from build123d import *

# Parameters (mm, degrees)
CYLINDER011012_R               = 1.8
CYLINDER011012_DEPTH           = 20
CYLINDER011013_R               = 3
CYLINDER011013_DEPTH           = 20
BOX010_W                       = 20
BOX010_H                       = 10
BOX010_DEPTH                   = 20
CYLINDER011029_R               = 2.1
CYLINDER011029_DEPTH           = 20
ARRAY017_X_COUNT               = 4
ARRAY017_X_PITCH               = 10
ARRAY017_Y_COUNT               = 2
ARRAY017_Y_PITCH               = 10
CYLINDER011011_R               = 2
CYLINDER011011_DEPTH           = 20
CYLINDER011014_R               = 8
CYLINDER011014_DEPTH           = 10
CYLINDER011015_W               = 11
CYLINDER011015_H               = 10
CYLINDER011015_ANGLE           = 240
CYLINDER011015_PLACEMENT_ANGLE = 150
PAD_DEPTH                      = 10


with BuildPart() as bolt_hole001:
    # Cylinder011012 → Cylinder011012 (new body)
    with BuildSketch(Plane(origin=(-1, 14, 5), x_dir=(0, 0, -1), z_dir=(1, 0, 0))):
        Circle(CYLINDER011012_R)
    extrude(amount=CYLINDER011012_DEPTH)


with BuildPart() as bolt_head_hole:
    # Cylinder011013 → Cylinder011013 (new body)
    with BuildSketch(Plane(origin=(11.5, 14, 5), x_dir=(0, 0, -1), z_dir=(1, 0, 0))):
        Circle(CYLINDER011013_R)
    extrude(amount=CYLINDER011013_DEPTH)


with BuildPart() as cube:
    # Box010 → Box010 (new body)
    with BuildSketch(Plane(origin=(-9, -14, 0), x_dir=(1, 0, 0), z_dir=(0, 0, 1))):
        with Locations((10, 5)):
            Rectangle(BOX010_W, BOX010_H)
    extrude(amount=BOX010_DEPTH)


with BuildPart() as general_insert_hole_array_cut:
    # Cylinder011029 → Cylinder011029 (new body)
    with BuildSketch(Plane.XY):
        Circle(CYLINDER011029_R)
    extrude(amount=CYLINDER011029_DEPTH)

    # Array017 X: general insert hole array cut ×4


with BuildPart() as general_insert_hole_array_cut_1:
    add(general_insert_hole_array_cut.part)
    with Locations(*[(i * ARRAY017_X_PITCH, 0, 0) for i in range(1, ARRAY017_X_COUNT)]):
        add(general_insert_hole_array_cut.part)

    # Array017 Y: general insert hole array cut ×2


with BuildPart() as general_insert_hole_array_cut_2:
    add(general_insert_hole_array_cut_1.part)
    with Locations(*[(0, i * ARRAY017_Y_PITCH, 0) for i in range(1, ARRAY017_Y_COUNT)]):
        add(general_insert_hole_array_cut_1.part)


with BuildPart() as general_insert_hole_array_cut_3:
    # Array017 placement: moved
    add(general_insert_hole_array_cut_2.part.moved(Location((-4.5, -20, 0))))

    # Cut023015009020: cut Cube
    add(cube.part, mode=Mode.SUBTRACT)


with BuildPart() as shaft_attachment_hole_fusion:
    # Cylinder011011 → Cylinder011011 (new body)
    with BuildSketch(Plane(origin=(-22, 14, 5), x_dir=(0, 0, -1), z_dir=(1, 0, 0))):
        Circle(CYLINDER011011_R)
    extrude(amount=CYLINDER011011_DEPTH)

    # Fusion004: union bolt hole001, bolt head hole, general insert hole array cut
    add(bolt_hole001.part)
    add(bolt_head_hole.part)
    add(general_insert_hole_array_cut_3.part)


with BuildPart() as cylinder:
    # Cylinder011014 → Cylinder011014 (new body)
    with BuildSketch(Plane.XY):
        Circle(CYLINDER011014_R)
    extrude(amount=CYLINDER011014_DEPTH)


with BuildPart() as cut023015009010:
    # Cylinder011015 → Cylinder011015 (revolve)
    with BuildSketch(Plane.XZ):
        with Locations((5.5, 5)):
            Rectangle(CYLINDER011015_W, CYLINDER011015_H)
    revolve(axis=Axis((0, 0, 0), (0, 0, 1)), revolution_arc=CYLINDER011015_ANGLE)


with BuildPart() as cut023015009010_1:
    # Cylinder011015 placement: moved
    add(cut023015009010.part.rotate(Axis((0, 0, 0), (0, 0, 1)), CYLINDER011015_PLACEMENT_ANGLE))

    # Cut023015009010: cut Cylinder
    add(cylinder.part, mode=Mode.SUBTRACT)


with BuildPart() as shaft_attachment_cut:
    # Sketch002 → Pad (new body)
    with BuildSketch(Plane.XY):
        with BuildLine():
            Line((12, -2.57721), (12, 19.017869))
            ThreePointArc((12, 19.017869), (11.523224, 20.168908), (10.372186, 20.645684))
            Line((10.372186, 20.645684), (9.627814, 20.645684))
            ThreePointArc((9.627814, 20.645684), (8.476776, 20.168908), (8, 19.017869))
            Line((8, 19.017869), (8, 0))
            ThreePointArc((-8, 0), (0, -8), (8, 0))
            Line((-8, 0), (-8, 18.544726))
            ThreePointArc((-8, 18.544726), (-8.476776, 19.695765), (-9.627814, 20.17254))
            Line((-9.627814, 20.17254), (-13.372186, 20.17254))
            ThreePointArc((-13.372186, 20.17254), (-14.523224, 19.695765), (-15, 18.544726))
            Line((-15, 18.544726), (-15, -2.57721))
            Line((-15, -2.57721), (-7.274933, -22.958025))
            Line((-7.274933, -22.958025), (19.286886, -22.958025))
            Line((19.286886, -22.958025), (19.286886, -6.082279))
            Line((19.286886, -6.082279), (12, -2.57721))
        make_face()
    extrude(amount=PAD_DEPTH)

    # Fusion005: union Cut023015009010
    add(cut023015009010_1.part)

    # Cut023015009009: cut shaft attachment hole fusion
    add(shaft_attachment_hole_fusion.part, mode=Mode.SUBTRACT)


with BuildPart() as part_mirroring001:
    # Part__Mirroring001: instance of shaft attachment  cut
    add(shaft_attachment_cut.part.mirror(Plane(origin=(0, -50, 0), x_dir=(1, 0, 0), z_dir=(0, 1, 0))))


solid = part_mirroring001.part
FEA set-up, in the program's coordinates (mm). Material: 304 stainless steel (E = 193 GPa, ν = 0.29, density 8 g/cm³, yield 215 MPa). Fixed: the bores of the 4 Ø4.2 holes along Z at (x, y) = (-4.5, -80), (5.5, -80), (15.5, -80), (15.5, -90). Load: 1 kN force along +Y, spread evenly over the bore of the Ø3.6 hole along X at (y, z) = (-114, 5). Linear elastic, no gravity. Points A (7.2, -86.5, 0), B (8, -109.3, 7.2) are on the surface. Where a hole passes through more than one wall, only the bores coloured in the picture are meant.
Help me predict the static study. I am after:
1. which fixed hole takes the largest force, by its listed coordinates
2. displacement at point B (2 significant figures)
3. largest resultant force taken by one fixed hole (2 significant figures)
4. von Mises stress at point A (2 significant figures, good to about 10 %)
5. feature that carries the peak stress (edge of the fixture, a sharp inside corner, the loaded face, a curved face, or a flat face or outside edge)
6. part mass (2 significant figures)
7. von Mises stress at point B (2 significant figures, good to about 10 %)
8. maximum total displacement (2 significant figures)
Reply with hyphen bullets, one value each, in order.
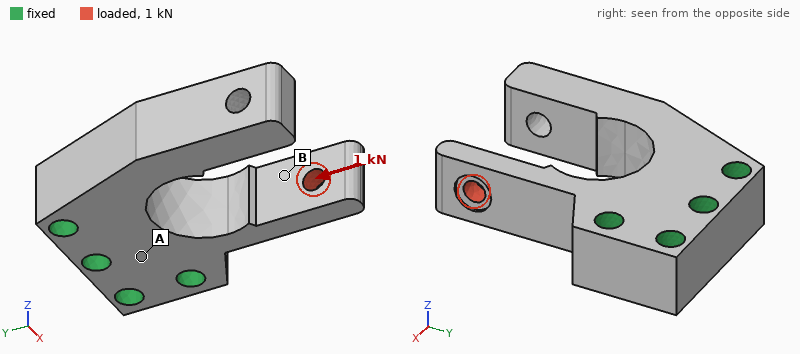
- (15.5, -90)
- 3.5 µm
- 480 N
- 6.1 MPa
- the loaded face
- 59 g
- 35 MPa
- 7.1 µm
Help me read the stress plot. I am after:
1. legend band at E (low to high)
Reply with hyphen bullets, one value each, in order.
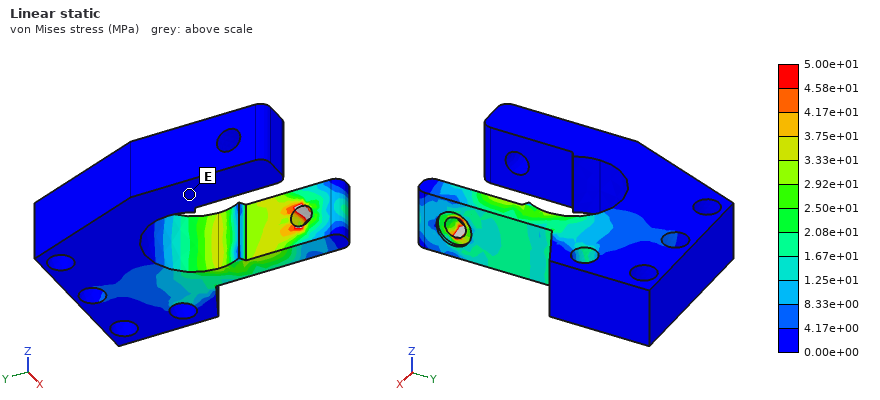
- 0.00e+00 to 4.17e+00 MPa
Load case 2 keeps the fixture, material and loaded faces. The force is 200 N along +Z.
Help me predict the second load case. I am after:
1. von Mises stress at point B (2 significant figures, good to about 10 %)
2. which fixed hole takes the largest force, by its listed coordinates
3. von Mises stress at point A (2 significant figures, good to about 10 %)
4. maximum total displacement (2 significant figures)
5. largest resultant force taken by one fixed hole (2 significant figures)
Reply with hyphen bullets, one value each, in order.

- 13 MPa
- (15.5, -90)
- 7.8 MPa
- 17 µm
- 280 N
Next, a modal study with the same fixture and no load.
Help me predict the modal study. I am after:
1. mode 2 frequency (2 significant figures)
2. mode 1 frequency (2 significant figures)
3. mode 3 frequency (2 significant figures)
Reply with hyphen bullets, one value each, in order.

- 5700 Hz
- 5600 Hz
- 5700 Hz
